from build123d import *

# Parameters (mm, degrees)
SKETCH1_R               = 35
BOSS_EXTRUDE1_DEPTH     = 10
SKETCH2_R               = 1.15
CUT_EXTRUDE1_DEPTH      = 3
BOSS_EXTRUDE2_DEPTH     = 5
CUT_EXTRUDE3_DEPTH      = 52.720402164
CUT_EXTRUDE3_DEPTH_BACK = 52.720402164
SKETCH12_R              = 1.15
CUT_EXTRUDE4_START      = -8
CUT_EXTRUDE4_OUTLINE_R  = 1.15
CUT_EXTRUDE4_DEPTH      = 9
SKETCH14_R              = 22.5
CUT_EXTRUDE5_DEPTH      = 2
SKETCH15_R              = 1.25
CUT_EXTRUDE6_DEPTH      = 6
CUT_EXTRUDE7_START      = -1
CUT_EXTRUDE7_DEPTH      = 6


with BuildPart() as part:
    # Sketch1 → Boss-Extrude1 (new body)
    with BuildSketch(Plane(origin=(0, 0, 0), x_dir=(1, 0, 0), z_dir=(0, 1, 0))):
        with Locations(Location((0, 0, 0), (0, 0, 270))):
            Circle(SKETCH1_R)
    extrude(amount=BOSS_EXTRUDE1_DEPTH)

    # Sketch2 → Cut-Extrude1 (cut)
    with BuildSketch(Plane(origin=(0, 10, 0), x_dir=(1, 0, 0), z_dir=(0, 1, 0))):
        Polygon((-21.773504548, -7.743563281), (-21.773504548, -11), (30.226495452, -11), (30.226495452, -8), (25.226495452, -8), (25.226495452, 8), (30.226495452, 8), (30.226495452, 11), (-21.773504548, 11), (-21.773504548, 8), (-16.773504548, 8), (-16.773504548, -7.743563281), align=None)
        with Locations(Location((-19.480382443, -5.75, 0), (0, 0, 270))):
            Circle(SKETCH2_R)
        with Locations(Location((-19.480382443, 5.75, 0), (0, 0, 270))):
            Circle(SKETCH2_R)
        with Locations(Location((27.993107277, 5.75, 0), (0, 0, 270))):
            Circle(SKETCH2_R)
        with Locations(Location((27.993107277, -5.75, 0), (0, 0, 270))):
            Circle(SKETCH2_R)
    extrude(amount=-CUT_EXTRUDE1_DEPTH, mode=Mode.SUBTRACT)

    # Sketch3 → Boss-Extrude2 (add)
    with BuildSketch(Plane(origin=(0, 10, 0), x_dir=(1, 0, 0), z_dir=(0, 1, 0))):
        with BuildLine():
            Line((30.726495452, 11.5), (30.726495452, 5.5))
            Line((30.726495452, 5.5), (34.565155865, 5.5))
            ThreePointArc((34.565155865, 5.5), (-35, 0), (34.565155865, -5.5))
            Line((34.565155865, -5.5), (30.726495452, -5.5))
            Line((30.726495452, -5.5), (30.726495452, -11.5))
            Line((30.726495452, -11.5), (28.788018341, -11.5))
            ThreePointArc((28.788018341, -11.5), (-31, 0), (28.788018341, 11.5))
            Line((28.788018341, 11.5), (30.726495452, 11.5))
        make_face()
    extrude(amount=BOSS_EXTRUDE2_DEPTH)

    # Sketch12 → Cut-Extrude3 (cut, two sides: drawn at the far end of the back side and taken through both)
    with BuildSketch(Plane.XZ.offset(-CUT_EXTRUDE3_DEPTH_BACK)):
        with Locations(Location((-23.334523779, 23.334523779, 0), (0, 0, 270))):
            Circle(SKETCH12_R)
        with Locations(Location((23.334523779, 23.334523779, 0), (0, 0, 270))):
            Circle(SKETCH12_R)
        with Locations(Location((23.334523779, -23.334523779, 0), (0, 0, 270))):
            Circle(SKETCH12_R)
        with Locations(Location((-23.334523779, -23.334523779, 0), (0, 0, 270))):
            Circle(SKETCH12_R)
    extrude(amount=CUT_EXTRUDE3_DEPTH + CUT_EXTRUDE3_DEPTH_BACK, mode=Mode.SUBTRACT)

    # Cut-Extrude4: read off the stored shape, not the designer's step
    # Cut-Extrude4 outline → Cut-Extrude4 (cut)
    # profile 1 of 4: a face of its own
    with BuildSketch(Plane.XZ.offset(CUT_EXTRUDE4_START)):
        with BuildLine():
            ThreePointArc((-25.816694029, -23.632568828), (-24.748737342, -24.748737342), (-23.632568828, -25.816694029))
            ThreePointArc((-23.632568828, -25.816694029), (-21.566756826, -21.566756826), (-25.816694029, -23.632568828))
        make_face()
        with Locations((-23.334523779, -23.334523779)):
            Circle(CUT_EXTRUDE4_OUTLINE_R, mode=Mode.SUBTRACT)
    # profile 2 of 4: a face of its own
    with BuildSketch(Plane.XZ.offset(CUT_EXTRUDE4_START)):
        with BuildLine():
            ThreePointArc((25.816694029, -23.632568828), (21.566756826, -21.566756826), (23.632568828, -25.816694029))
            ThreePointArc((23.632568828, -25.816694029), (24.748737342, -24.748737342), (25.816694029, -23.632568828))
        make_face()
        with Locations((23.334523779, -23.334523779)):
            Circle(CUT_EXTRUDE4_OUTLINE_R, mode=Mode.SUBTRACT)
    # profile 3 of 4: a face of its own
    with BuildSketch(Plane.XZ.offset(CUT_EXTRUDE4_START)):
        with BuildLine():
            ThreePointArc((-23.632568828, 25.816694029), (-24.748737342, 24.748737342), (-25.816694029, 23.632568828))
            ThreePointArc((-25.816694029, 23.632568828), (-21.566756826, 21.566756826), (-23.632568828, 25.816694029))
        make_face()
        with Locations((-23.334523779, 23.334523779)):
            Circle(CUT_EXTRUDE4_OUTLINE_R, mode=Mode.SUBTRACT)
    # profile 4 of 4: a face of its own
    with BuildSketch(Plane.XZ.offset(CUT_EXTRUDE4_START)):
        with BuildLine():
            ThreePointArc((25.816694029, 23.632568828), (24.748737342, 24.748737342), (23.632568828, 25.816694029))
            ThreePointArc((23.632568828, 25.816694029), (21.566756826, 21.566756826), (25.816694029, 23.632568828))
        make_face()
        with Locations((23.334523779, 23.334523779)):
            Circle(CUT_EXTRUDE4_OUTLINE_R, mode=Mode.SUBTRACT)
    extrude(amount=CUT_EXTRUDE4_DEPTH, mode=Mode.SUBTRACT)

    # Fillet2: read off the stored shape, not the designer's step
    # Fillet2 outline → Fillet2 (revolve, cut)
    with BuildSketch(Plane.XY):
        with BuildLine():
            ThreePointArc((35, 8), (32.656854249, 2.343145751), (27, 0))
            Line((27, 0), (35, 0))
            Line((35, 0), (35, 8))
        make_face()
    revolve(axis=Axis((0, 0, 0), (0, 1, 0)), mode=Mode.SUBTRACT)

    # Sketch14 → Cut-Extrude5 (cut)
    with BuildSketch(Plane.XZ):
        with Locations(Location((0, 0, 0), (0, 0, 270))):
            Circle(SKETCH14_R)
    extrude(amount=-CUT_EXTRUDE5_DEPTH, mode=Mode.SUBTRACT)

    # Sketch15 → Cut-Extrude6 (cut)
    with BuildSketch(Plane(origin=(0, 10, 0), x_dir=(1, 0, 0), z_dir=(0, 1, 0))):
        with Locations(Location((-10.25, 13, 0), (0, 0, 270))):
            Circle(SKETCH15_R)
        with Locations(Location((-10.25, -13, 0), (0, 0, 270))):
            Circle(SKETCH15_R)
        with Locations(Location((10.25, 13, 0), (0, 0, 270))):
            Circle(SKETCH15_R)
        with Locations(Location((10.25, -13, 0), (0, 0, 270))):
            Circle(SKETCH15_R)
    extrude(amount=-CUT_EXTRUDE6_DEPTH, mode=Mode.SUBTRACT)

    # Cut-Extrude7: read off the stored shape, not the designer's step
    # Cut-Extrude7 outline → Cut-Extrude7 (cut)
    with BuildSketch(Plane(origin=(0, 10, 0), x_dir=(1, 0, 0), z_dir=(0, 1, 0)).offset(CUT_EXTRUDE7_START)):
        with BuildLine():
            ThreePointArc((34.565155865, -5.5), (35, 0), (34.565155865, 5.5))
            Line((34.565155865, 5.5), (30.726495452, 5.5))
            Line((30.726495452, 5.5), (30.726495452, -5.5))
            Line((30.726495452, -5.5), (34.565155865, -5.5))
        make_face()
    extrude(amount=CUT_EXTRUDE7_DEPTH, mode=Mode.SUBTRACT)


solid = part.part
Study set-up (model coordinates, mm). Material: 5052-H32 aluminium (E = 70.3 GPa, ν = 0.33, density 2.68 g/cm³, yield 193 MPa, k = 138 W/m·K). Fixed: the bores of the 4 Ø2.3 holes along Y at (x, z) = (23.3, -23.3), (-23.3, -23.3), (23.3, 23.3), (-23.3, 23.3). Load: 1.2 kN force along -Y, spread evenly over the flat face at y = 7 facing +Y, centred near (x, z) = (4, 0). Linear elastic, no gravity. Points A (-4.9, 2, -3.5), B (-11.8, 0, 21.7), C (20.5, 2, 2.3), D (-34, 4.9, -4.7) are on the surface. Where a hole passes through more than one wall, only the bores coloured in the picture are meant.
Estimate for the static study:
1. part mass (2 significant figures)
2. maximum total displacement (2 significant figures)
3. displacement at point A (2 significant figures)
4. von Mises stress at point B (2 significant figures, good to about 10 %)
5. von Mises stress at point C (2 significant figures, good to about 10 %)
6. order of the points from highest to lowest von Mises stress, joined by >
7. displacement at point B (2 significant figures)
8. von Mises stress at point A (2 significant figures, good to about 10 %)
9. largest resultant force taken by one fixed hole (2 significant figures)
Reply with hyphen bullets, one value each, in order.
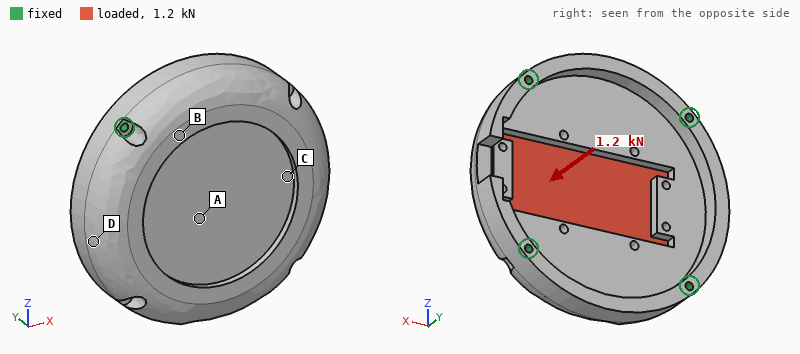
- 87 g
- 15 µm
- 13 µm
- 5.9 MPa
- 11 MPa
- A > C > B > D
- 4.1 µm
- 15 MPa
- 600 N
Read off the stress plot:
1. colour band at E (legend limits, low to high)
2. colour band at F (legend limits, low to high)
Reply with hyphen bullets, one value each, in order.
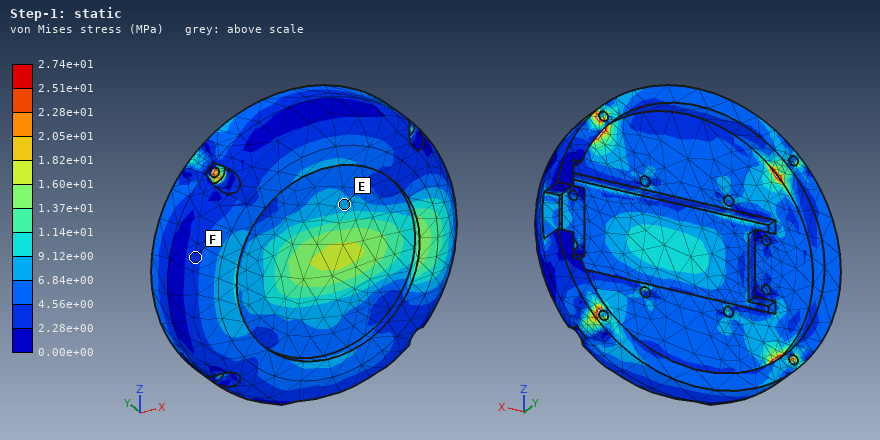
- 6.84e+00 to 9.12e+00 MPa
- 2.28e+00 to 4.56e+00 MPa
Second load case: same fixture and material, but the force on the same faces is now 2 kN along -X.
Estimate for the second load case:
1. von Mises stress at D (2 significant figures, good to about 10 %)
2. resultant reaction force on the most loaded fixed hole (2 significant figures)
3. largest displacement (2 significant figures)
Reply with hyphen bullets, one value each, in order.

- 3.1 MPa
- 520 N
- 4.0 µm
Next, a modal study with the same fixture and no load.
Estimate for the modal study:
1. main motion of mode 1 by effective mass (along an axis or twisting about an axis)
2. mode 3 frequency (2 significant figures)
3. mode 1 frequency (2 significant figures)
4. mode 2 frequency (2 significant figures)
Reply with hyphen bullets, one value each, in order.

- along Y
- 14 kHz
- 10 kHz
- 14 kHz
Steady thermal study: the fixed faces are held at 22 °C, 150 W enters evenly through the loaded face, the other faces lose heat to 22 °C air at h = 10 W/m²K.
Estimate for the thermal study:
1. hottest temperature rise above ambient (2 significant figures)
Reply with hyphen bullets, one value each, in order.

- 53 K
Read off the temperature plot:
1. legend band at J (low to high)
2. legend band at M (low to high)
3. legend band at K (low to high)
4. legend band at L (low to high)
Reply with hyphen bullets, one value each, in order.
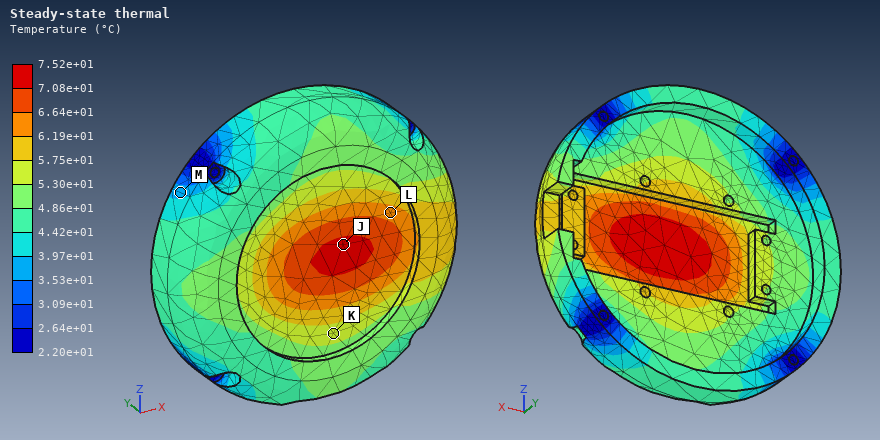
- 7.08e+01 to 7.52e+01 °C
- 3.53e+01 to 3.97e+01 °C
- 5.30e+01 to 5.75e+01 °C
- 6.19e+01 to 6.64e+01 °C
